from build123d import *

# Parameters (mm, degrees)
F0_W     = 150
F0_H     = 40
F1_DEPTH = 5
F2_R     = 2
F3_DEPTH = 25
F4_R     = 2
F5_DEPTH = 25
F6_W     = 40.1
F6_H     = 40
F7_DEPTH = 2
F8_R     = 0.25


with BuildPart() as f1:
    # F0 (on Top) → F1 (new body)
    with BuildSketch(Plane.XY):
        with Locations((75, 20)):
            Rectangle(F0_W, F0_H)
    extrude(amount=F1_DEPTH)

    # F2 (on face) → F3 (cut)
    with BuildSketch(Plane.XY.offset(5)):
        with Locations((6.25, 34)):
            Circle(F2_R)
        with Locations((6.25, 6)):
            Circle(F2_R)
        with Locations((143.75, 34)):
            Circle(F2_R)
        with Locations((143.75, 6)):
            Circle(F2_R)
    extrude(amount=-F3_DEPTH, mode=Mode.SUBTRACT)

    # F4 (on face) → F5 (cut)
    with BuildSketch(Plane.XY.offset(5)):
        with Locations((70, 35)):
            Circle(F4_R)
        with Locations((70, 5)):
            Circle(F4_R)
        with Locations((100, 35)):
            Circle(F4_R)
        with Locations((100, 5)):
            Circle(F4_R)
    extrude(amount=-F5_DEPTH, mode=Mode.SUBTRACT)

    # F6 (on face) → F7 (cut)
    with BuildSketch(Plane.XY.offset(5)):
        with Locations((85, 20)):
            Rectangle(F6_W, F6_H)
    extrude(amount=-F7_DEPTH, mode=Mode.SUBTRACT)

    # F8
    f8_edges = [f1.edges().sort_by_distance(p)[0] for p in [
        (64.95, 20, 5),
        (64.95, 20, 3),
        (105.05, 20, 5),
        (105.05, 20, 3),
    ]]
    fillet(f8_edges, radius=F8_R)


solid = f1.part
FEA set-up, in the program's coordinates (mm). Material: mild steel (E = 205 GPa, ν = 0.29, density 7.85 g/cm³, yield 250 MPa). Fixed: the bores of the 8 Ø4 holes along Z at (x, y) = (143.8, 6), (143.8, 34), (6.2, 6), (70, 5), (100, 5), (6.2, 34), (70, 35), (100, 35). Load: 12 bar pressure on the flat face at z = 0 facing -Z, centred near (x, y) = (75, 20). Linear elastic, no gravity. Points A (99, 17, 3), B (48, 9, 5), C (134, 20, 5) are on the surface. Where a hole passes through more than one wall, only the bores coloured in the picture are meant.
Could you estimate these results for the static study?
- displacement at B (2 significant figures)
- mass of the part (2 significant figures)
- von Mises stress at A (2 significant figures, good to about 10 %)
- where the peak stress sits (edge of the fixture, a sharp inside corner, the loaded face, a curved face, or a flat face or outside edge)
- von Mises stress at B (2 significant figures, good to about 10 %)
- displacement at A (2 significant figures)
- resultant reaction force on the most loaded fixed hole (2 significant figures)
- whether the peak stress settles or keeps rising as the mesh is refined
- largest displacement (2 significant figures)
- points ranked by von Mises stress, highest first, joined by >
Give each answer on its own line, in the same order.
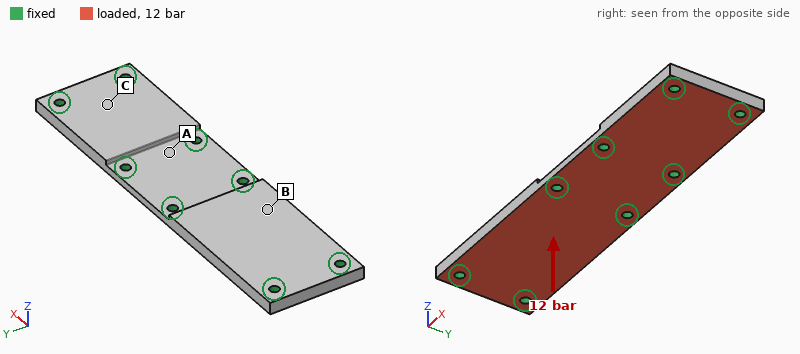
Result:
32 µm
210 g
31 MPa
edge of the fixture
54 MPa
6.0 µm
1.1 kN
keeps rising
37 µm
B > A > C
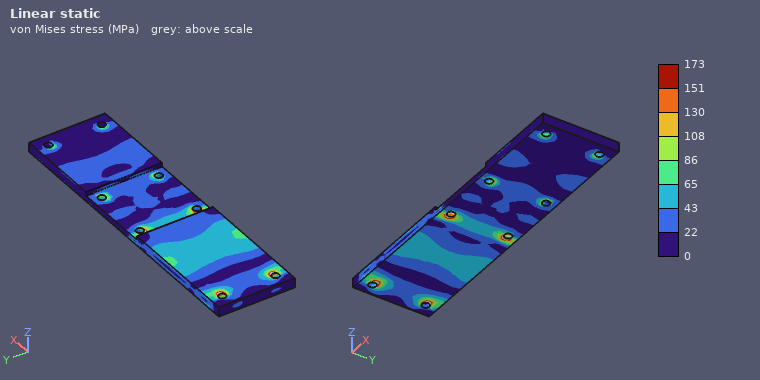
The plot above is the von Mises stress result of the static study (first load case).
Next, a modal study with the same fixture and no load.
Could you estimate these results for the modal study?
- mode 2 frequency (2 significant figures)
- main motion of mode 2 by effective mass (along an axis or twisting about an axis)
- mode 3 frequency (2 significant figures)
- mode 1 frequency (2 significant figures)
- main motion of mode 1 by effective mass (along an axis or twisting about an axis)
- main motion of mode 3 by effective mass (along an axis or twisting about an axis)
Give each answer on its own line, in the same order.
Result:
8300 Hz
twisting about X
10 kHz
5200 Hz
along Z
along Z
